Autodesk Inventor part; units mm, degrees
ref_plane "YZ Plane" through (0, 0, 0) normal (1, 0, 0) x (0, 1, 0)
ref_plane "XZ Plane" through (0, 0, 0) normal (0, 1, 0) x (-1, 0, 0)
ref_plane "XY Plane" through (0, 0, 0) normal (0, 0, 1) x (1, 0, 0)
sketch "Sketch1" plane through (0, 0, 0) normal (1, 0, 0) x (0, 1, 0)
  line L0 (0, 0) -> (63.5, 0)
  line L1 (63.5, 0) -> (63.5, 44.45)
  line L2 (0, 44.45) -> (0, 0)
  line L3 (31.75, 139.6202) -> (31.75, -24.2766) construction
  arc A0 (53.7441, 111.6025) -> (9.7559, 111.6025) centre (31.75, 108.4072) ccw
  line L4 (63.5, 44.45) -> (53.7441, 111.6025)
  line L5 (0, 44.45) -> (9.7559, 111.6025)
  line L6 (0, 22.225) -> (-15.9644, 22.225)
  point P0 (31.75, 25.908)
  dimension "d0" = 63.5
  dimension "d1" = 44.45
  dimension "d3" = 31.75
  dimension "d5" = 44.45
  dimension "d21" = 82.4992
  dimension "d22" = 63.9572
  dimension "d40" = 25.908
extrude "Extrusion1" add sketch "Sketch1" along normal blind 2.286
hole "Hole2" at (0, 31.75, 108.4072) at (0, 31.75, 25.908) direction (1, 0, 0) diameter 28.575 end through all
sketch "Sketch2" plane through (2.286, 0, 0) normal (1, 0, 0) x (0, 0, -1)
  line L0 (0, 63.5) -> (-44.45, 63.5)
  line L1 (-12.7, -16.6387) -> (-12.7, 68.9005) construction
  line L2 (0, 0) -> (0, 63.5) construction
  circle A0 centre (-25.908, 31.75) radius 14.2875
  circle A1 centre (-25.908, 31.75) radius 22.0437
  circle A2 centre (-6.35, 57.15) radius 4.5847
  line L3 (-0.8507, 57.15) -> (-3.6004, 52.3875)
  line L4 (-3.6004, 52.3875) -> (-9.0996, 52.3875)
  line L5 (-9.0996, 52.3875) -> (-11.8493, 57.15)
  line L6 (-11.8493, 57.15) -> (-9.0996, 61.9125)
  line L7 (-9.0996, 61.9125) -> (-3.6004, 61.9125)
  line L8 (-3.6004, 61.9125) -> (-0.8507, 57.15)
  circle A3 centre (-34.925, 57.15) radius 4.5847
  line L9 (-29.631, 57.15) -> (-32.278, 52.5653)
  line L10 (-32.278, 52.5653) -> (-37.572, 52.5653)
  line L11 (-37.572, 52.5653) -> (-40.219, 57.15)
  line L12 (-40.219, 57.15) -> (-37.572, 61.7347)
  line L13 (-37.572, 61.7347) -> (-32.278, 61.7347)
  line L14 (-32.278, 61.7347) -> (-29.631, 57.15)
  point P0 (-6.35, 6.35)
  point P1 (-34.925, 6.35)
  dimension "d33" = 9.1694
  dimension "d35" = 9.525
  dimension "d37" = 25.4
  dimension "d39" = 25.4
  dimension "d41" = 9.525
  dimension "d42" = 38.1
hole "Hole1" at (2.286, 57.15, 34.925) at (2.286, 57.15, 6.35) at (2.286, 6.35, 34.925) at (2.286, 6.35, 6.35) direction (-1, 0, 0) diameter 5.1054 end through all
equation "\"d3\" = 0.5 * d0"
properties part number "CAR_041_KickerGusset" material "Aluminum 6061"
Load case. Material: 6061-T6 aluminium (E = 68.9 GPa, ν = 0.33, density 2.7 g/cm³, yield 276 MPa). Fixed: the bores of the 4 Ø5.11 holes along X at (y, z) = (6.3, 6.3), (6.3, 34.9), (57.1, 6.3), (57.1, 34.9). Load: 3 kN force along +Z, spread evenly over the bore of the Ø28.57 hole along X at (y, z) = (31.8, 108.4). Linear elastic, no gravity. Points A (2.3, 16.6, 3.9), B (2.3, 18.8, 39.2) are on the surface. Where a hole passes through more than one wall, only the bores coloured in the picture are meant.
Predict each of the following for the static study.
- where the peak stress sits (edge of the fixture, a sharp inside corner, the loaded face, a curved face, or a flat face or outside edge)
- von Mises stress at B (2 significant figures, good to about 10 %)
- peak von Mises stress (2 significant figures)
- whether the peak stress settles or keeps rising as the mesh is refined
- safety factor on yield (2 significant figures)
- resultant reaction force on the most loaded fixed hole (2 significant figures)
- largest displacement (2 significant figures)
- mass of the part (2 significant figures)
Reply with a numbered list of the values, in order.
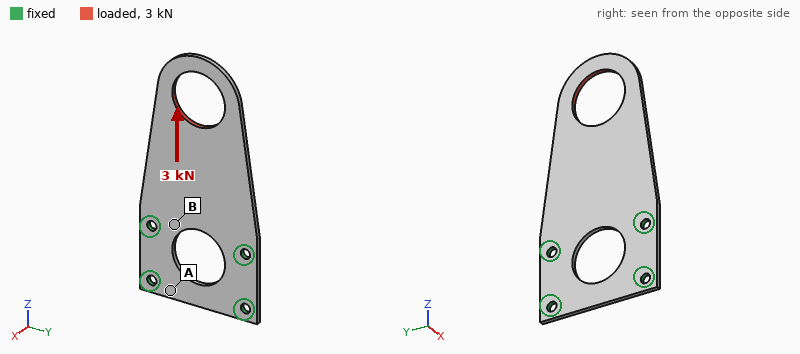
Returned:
1. the loaded face
2. 22 MPa
3. 110 MPa
4. settles
5. 2.5
6. 1.4 kN
7. 69 µm
8. 35 g
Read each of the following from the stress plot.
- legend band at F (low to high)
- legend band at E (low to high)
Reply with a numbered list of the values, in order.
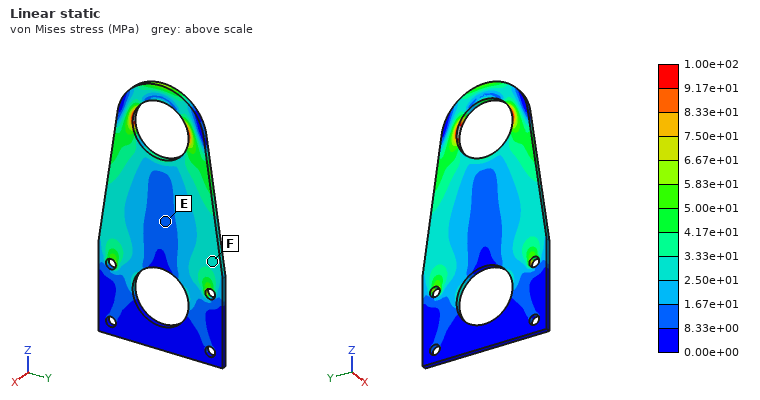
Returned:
1. 2.50e+01 to 3.33e+01 MPa
2. 8.33e+00 to 1.67e+01 MPa
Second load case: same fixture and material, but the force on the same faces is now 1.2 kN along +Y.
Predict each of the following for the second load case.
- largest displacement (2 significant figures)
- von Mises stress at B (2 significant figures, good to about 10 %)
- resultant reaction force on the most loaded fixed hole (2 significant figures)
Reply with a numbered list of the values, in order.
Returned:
1. 0.17 mm
2. 16 MPa
3. 1.7 kN
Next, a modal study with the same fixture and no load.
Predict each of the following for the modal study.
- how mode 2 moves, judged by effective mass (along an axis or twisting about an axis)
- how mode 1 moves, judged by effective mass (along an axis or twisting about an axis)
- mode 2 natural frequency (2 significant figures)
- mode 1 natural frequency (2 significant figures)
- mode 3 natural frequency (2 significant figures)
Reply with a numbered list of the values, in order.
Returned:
1. twisting about Z
2. along X
3. 1100 Hz
4. 290 Hz
5. 1300 Hz
